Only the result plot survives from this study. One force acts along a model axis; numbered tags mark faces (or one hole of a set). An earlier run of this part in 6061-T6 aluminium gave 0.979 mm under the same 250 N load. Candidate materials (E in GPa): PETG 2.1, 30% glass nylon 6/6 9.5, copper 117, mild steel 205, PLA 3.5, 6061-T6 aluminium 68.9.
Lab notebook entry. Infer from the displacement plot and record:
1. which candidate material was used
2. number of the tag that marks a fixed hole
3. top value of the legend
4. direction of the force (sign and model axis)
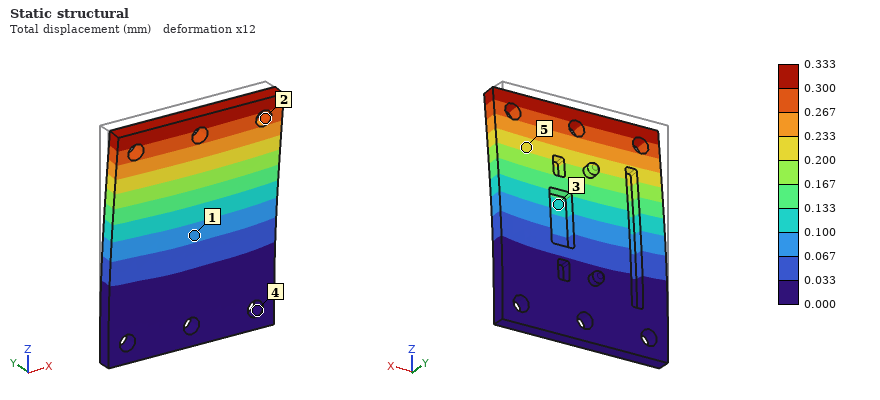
mild steel
4
0.333 mm
-Y
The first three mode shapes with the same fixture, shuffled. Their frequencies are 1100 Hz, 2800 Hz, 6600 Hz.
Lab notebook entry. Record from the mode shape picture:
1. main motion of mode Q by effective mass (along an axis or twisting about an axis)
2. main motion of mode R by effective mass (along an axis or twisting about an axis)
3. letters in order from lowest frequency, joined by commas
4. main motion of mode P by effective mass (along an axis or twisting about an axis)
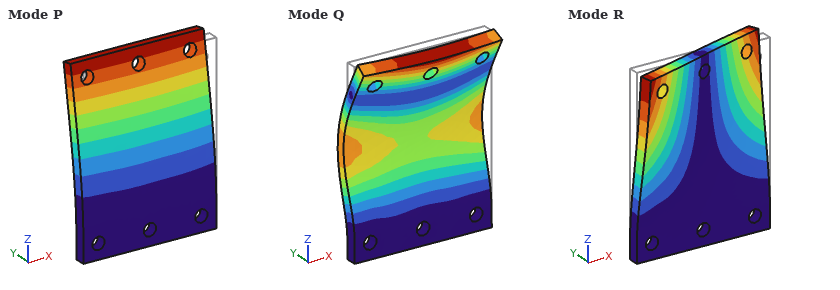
along Y
twisting about Z
P, R, Q
along Y
